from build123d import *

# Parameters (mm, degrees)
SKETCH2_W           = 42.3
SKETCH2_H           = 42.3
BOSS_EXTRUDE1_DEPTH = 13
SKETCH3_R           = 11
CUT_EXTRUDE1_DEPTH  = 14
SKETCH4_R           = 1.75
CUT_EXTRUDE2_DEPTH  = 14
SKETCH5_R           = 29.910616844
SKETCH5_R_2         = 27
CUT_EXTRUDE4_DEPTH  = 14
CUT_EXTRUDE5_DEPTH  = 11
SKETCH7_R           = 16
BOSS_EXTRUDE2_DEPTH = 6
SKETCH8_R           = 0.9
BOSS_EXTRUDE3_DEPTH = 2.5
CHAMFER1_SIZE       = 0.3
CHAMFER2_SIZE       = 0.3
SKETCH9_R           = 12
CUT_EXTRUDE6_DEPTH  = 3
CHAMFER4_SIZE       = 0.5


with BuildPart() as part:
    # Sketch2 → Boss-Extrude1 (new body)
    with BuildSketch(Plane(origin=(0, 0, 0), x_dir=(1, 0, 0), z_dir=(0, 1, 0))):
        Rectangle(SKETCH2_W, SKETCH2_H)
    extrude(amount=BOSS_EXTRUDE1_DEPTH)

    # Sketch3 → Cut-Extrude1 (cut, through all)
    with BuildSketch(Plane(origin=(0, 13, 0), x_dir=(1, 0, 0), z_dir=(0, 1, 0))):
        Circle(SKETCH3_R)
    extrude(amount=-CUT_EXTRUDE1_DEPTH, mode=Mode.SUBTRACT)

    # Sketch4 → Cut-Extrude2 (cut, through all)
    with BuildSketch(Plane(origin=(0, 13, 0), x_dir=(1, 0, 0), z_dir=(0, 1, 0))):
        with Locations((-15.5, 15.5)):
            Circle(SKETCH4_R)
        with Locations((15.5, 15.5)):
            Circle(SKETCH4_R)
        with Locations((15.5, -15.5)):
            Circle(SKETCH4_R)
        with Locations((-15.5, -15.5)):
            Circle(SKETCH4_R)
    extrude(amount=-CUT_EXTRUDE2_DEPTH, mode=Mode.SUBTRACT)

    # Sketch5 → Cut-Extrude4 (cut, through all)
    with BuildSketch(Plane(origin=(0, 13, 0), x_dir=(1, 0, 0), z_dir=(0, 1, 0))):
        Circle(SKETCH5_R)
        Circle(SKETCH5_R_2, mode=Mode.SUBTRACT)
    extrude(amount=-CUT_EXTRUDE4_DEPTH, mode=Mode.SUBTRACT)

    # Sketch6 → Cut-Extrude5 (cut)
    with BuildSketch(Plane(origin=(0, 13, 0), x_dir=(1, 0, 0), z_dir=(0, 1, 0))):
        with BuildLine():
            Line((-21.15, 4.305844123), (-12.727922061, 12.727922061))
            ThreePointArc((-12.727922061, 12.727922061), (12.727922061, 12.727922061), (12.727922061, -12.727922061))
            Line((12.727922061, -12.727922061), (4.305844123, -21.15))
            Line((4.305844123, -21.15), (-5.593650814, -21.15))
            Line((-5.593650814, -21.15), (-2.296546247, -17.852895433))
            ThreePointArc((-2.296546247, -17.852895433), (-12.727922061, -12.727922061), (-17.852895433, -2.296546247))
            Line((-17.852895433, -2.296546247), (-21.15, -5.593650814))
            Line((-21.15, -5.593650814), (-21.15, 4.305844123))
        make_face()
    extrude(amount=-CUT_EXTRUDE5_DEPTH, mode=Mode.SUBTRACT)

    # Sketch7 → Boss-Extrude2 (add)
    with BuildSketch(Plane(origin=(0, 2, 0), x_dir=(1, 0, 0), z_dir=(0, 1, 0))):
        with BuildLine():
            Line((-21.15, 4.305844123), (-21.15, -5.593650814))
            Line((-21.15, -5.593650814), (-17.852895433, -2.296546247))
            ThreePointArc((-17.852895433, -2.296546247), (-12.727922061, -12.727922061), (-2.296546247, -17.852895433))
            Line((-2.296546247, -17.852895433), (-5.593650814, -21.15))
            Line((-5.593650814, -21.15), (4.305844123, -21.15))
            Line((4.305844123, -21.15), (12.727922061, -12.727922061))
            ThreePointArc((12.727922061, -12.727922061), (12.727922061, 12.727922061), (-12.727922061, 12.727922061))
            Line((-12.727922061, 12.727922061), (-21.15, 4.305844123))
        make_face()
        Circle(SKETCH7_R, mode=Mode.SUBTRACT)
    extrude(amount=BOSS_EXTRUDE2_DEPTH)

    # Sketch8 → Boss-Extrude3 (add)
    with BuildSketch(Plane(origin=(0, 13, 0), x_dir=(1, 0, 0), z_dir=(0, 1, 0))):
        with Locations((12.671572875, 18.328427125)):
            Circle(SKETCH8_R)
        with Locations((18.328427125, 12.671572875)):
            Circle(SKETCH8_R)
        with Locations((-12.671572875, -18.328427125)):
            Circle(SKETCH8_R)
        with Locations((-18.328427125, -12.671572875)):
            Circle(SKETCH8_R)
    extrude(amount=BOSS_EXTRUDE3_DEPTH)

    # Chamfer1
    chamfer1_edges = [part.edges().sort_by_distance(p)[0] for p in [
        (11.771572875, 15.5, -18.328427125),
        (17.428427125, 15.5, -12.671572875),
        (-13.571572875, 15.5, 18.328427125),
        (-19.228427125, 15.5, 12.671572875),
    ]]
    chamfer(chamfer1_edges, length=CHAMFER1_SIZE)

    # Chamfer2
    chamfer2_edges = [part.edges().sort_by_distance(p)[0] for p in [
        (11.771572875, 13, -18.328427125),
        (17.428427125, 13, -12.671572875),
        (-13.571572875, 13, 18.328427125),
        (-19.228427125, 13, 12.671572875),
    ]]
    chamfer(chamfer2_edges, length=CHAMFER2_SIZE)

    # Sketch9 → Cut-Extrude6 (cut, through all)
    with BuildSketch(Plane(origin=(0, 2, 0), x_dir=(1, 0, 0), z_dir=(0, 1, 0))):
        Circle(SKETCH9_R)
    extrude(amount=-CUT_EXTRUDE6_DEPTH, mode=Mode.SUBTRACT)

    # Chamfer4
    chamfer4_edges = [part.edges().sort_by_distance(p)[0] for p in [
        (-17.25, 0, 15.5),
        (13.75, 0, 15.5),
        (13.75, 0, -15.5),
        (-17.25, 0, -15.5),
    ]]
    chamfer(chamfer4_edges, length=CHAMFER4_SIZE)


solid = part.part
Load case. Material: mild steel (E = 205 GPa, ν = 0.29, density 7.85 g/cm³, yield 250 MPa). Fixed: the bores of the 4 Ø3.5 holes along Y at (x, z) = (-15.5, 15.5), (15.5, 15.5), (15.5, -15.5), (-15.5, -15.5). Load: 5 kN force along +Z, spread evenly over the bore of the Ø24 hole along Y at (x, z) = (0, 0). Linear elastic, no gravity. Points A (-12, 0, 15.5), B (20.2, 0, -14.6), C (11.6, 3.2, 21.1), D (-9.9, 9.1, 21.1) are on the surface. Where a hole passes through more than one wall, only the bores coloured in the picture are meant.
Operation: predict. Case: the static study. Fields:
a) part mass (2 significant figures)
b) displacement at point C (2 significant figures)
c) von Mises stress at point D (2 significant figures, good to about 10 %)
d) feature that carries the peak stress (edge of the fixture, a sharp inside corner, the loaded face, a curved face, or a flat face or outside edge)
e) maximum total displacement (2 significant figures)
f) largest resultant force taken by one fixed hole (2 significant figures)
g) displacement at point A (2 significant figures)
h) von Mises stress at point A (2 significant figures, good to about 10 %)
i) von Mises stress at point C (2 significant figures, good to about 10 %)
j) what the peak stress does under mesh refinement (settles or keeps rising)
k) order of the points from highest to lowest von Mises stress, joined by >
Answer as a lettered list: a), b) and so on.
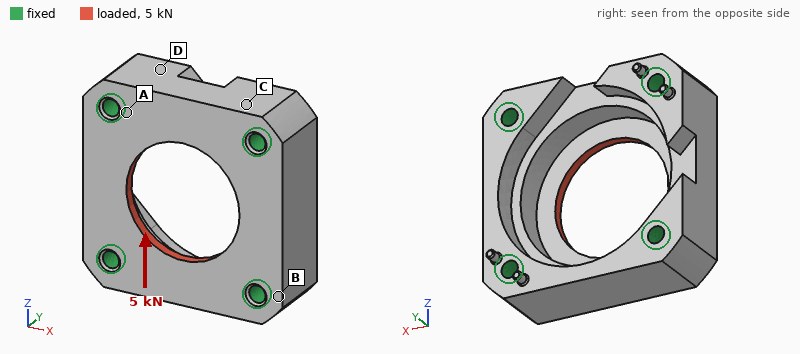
a) 87 g
b) 1.0 µm
c) 12 MPa
d) edge of the fixture
e) 5.0 µm
f) 1.3 kN
g) 0.80 µm
h) 36 MPa
i) 19 MPa
j) keeps rising
k) A > C > D > B
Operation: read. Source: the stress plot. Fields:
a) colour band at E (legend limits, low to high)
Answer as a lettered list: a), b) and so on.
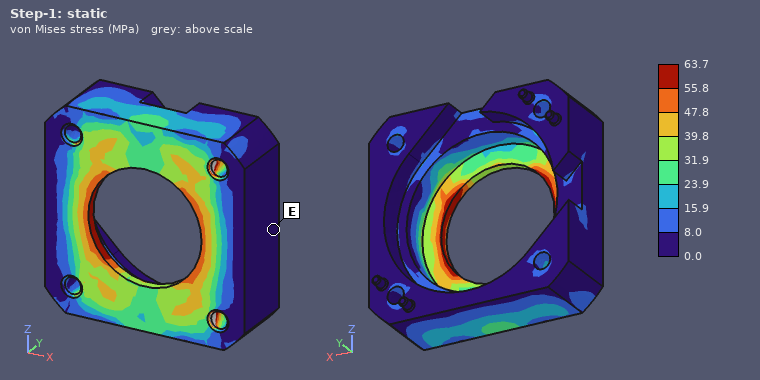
a) 0.0 to 8.0 MPa
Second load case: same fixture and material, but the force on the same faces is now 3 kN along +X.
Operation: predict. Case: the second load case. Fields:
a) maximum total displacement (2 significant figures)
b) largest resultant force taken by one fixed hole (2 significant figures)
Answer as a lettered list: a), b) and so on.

a) 3.0 µm
b) 760 N
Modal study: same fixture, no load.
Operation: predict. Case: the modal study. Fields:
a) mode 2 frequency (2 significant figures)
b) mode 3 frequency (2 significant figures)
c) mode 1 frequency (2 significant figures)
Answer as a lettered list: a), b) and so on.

a) 40 kHz
b) 40 kHz
c) 32 kHz
